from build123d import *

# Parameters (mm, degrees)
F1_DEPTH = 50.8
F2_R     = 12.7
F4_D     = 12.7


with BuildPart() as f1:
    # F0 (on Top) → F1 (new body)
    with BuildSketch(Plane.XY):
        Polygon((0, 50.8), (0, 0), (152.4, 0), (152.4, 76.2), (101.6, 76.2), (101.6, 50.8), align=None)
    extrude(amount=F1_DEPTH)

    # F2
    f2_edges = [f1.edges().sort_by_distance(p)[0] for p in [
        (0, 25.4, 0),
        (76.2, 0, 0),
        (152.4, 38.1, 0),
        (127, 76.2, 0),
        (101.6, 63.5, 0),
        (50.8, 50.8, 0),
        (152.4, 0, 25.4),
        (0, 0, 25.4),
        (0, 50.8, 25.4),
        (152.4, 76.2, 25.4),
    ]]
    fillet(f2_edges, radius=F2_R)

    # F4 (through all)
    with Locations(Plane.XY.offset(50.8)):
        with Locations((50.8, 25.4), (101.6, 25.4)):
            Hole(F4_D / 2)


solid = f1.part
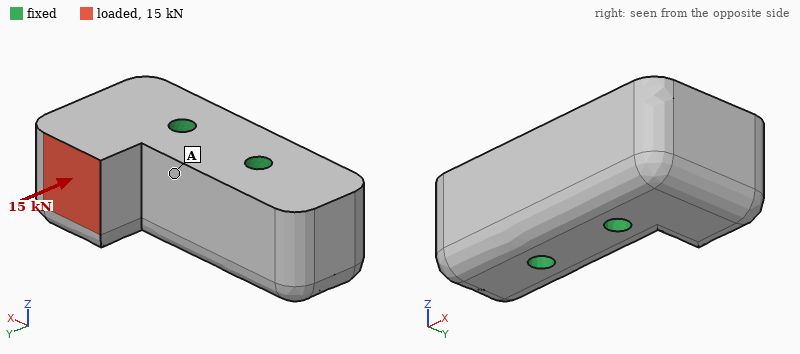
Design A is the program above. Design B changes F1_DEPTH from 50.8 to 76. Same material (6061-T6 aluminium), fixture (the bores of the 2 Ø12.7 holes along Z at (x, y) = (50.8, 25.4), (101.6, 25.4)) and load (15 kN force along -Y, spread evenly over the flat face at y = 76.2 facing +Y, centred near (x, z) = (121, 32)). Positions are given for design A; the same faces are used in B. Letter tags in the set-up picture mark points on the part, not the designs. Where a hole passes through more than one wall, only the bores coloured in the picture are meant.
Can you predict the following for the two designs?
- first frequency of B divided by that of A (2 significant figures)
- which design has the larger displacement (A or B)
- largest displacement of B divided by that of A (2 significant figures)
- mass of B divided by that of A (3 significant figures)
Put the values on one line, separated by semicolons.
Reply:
1.0; A; 0.64; 1.51
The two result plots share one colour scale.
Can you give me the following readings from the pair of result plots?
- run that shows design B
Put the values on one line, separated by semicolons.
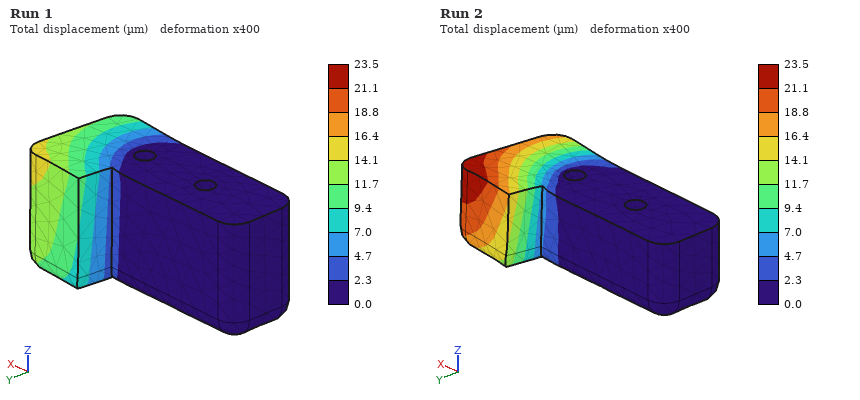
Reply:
Run 1
